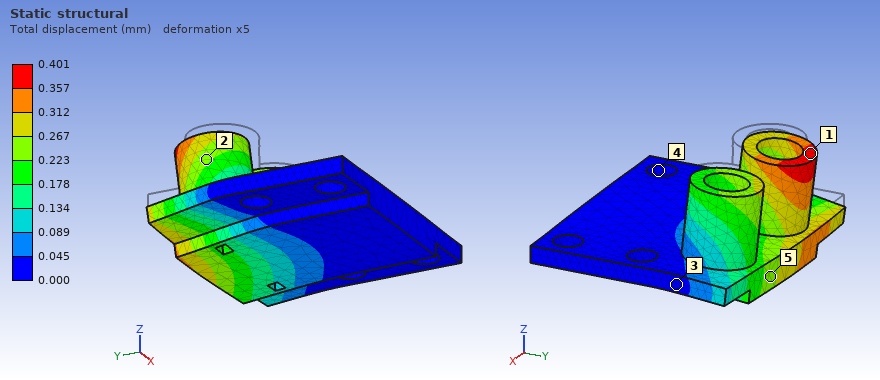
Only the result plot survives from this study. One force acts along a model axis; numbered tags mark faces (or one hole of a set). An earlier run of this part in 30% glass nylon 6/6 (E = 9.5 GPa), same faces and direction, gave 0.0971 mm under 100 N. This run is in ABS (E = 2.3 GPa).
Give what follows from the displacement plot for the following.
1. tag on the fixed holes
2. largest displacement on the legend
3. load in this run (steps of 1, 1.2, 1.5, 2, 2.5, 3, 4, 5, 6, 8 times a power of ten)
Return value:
4
0.401 mm
100 N
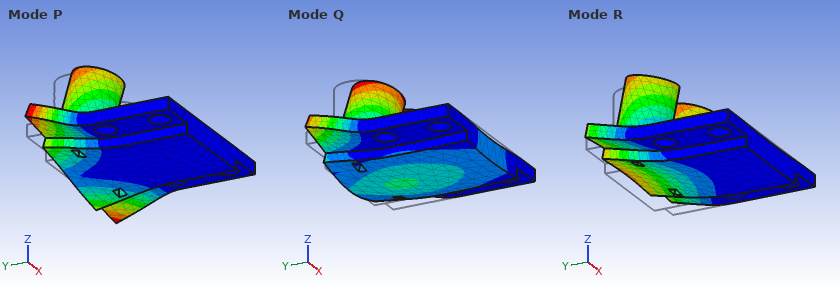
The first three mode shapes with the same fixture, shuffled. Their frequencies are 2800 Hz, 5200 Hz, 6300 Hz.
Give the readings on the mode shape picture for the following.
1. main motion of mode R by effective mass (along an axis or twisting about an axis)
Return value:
along Z
